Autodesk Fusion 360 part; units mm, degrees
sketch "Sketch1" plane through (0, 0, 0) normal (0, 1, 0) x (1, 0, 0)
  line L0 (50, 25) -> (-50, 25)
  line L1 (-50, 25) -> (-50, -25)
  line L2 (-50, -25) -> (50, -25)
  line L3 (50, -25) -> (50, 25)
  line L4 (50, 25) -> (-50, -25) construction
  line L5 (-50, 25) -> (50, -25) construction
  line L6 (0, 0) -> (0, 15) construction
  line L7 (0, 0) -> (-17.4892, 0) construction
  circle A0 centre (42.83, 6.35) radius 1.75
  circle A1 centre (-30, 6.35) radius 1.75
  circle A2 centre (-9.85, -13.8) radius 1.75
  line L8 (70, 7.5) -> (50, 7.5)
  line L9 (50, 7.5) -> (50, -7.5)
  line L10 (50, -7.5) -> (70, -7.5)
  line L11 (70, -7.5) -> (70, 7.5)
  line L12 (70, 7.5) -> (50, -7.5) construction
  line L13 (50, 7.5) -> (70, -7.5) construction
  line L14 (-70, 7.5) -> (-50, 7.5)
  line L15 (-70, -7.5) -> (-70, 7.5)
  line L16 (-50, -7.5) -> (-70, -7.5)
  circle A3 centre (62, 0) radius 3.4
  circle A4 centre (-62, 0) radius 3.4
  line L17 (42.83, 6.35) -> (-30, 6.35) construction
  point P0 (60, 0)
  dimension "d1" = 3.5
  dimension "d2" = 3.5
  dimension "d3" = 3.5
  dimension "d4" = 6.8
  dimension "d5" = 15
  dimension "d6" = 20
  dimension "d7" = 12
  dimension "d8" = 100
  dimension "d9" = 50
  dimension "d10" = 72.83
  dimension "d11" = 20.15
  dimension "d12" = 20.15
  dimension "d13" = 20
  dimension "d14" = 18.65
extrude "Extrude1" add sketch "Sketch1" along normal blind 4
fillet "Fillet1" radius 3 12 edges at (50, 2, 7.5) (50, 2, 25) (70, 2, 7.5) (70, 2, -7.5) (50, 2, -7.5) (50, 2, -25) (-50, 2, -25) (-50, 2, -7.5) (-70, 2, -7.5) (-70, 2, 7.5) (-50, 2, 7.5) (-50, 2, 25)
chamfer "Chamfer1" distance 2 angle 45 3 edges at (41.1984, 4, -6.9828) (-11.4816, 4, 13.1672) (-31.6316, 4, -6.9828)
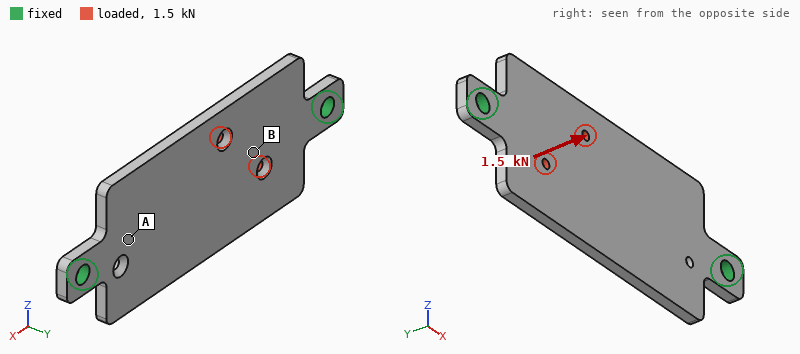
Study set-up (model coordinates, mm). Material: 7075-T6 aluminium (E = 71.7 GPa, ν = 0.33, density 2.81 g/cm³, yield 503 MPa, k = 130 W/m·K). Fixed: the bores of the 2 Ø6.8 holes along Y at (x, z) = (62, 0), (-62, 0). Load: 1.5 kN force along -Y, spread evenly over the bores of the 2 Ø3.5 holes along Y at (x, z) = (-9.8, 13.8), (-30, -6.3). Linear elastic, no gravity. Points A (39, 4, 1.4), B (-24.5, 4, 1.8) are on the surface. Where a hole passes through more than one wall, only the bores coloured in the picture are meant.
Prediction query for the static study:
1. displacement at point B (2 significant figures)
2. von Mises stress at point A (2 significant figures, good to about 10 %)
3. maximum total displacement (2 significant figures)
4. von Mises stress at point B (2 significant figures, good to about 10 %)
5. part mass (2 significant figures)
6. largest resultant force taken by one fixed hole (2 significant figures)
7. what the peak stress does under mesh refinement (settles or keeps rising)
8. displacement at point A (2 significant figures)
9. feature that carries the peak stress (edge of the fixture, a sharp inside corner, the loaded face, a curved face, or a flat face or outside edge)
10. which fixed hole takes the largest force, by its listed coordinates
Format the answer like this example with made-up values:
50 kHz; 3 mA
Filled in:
0.74 mm; 41 MPa; 1.2 mm; 130 MPa; 61 g; 1.1 kN; keeps rising; 0.28 mm; edge of the fixture; (-62, 0)
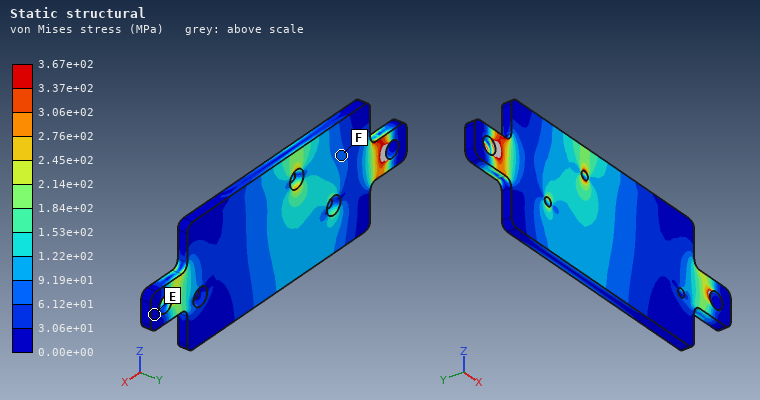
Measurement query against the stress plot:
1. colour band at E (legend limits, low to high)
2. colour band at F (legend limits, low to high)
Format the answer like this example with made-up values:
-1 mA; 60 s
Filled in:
0.00e+00 to 3.06e+01 MPa; 6.12e+01 to 9.19e+01 MPa
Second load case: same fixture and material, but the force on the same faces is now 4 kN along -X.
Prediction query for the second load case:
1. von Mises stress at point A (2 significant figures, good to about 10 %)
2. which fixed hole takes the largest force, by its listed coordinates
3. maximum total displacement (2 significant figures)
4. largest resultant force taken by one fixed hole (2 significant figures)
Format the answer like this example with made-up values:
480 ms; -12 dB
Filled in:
18 MPa; (-62, 0); 58 µm; 2.4 kN
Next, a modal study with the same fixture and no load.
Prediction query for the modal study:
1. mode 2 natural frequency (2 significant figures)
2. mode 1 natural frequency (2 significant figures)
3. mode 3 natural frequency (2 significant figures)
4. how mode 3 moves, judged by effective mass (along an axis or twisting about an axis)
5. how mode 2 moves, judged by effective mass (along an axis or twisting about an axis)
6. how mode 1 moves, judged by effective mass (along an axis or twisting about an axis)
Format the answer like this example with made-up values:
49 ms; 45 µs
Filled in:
1400 Hz; 1100 Hz; 3100 Hz; twisting about Z; twisting about X; along Y
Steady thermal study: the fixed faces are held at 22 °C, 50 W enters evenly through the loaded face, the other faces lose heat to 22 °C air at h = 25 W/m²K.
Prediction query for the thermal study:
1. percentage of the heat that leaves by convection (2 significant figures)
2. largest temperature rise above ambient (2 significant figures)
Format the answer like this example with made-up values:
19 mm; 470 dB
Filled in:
26 %; 82 K
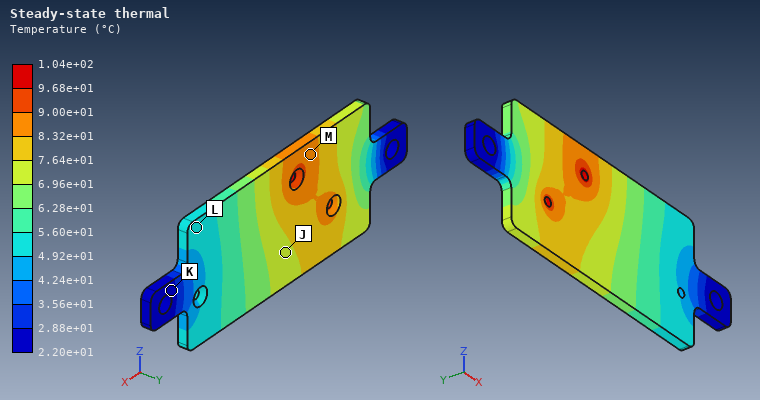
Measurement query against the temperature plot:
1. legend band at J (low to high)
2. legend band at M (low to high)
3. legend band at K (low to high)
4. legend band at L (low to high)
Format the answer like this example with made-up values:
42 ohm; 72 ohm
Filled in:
6.96e+01 to 7.64e+01 °C; 8.32e+01 to 9.00e+01 °C; 2.20e+01 to 2.88e+01 °C; 4.92e+01 to 5.60e+01 °C
